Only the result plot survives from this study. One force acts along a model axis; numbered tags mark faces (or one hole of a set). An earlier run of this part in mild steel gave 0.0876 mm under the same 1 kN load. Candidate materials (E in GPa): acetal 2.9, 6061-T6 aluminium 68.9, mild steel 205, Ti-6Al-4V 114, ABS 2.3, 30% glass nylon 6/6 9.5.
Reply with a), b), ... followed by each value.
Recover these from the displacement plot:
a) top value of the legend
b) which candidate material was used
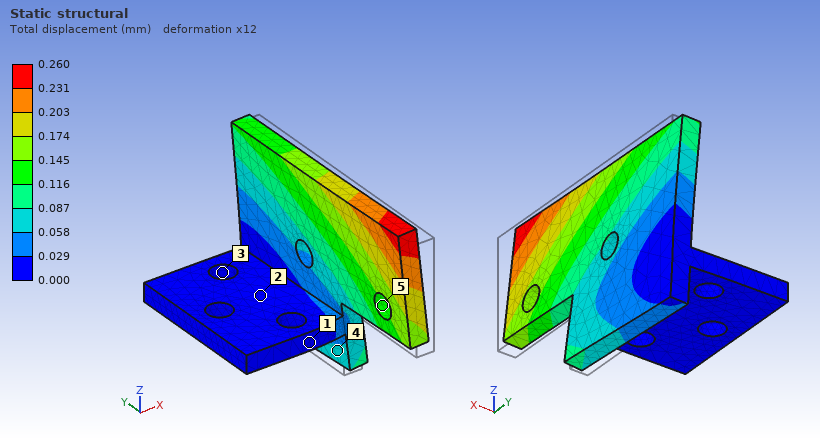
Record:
a) 0.260 mm
b) 6061-T6 aluminium
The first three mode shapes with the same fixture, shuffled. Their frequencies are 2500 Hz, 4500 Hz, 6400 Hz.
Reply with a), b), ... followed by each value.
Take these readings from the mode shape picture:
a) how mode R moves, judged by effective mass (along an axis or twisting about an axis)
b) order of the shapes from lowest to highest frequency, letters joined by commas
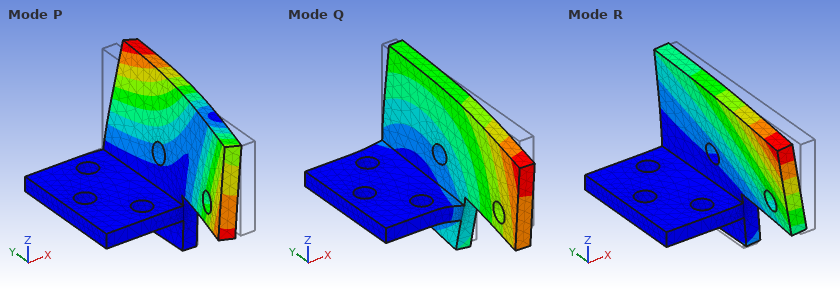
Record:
a) along X
b) R, P, Q
